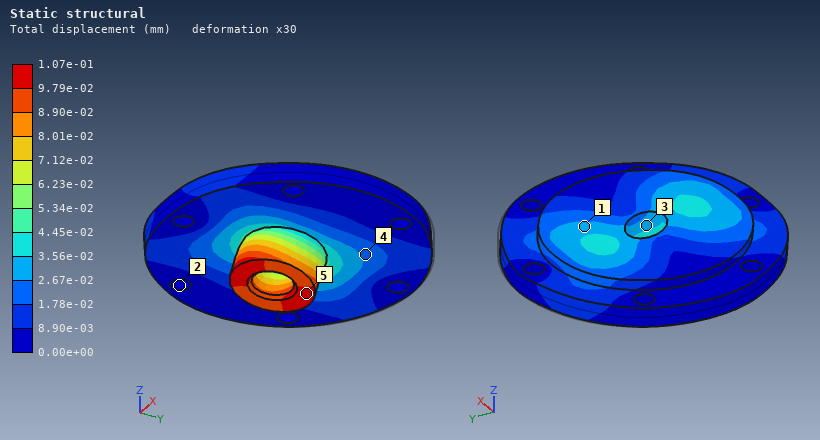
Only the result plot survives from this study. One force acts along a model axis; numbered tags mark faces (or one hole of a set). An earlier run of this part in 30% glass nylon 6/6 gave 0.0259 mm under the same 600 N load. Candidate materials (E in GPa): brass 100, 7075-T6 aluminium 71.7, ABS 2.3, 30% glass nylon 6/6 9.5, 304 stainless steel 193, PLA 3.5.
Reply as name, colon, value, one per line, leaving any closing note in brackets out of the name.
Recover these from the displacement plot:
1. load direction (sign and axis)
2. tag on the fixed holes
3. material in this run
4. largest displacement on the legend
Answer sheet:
load direction: -Y
tag on the fixed holes: 2
material in this run: ABS
largest displacement on the legend: 1.07e-01 mm
